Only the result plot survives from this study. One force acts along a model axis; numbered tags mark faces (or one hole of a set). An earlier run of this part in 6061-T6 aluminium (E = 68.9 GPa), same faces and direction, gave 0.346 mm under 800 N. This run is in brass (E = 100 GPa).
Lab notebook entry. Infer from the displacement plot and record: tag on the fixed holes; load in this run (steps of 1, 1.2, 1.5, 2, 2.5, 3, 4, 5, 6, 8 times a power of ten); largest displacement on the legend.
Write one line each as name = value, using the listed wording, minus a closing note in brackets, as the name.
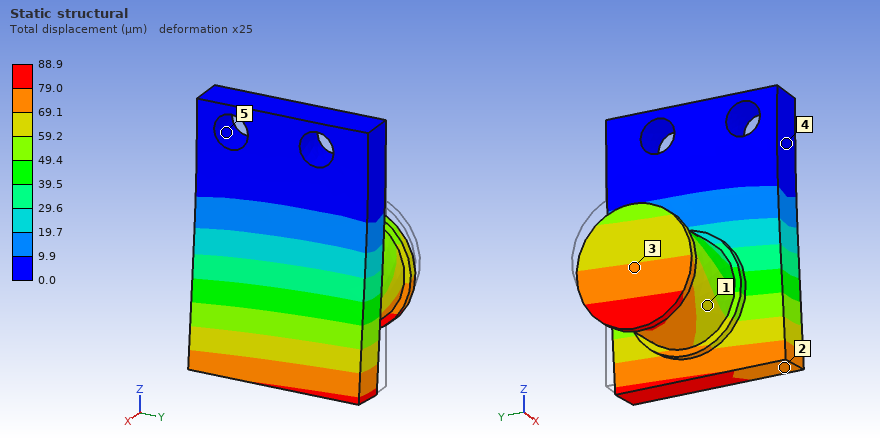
tag on the fixed holes = 5
load in this run = 300 N
largest displacement on the legend = 88.9 µm
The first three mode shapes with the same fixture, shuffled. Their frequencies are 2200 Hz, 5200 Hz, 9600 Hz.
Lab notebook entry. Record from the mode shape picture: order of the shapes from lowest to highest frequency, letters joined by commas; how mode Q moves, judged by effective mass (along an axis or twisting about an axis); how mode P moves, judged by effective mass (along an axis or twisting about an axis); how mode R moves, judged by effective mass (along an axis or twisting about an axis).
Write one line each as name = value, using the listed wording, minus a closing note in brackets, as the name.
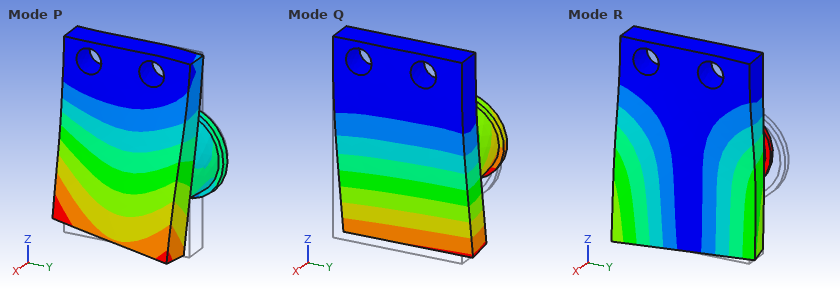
order of the shapes from lowest to highest frequency, letters joined by commas = Q, R, P
how mode Q moves, judged by effective mass = along X
how mode P moves, judged by effective mass = along Y
how mode R moves, judged by effective mass = along Y
